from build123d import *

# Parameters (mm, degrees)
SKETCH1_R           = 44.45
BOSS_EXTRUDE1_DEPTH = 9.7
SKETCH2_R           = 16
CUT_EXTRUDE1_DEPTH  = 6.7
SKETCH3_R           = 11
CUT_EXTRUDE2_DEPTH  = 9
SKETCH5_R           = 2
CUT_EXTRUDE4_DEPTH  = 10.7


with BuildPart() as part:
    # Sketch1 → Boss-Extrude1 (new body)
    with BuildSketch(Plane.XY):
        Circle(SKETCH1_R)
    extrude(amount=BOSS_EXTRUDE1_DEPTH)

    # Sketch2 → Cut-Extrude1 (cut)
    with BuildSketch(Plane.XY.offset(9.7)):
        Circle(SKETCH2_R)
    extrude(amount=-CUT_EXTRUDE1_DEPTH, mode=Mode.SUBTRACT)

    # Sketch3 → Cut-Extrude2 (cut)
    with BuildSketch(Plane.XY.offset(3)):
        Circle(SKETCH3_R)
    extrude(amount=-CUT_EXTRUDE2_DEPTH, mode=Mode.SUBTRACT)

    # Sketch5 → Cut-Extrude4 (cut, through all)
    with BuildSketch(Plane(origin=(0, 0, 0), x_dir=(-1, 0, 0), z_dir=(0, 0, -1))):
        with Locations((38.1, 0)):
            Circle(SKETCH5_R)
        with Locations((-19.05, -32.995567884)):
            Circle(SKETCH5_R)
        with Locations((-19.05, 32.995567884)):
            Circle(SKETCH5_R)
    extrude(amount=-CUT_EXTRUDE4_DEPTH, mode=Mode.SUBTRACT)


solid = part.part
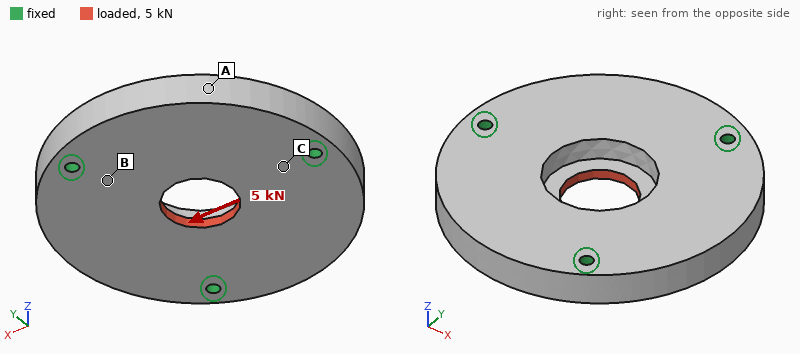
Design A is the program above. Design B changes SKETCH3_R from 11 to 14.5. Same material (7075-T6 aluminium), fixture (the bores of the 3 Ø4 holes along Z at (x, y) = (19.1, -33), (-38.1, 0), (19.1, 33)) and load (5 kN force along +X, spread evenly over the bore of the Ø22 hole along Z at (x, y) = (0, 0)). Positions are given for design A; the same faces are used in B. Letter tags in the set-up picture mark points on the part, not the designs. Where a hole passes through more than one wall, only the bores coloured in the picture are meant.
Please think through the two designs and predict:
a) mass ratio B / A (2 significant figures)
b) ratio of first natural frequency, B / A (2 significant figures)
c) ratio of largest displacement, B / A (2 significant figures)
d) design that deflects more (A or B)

0.98
1.00
0.82
A
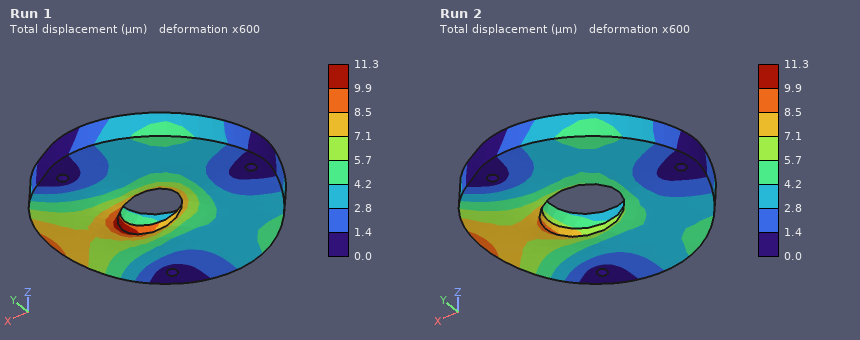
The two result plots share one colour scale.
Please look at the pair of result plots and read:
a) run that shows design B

Run 2
